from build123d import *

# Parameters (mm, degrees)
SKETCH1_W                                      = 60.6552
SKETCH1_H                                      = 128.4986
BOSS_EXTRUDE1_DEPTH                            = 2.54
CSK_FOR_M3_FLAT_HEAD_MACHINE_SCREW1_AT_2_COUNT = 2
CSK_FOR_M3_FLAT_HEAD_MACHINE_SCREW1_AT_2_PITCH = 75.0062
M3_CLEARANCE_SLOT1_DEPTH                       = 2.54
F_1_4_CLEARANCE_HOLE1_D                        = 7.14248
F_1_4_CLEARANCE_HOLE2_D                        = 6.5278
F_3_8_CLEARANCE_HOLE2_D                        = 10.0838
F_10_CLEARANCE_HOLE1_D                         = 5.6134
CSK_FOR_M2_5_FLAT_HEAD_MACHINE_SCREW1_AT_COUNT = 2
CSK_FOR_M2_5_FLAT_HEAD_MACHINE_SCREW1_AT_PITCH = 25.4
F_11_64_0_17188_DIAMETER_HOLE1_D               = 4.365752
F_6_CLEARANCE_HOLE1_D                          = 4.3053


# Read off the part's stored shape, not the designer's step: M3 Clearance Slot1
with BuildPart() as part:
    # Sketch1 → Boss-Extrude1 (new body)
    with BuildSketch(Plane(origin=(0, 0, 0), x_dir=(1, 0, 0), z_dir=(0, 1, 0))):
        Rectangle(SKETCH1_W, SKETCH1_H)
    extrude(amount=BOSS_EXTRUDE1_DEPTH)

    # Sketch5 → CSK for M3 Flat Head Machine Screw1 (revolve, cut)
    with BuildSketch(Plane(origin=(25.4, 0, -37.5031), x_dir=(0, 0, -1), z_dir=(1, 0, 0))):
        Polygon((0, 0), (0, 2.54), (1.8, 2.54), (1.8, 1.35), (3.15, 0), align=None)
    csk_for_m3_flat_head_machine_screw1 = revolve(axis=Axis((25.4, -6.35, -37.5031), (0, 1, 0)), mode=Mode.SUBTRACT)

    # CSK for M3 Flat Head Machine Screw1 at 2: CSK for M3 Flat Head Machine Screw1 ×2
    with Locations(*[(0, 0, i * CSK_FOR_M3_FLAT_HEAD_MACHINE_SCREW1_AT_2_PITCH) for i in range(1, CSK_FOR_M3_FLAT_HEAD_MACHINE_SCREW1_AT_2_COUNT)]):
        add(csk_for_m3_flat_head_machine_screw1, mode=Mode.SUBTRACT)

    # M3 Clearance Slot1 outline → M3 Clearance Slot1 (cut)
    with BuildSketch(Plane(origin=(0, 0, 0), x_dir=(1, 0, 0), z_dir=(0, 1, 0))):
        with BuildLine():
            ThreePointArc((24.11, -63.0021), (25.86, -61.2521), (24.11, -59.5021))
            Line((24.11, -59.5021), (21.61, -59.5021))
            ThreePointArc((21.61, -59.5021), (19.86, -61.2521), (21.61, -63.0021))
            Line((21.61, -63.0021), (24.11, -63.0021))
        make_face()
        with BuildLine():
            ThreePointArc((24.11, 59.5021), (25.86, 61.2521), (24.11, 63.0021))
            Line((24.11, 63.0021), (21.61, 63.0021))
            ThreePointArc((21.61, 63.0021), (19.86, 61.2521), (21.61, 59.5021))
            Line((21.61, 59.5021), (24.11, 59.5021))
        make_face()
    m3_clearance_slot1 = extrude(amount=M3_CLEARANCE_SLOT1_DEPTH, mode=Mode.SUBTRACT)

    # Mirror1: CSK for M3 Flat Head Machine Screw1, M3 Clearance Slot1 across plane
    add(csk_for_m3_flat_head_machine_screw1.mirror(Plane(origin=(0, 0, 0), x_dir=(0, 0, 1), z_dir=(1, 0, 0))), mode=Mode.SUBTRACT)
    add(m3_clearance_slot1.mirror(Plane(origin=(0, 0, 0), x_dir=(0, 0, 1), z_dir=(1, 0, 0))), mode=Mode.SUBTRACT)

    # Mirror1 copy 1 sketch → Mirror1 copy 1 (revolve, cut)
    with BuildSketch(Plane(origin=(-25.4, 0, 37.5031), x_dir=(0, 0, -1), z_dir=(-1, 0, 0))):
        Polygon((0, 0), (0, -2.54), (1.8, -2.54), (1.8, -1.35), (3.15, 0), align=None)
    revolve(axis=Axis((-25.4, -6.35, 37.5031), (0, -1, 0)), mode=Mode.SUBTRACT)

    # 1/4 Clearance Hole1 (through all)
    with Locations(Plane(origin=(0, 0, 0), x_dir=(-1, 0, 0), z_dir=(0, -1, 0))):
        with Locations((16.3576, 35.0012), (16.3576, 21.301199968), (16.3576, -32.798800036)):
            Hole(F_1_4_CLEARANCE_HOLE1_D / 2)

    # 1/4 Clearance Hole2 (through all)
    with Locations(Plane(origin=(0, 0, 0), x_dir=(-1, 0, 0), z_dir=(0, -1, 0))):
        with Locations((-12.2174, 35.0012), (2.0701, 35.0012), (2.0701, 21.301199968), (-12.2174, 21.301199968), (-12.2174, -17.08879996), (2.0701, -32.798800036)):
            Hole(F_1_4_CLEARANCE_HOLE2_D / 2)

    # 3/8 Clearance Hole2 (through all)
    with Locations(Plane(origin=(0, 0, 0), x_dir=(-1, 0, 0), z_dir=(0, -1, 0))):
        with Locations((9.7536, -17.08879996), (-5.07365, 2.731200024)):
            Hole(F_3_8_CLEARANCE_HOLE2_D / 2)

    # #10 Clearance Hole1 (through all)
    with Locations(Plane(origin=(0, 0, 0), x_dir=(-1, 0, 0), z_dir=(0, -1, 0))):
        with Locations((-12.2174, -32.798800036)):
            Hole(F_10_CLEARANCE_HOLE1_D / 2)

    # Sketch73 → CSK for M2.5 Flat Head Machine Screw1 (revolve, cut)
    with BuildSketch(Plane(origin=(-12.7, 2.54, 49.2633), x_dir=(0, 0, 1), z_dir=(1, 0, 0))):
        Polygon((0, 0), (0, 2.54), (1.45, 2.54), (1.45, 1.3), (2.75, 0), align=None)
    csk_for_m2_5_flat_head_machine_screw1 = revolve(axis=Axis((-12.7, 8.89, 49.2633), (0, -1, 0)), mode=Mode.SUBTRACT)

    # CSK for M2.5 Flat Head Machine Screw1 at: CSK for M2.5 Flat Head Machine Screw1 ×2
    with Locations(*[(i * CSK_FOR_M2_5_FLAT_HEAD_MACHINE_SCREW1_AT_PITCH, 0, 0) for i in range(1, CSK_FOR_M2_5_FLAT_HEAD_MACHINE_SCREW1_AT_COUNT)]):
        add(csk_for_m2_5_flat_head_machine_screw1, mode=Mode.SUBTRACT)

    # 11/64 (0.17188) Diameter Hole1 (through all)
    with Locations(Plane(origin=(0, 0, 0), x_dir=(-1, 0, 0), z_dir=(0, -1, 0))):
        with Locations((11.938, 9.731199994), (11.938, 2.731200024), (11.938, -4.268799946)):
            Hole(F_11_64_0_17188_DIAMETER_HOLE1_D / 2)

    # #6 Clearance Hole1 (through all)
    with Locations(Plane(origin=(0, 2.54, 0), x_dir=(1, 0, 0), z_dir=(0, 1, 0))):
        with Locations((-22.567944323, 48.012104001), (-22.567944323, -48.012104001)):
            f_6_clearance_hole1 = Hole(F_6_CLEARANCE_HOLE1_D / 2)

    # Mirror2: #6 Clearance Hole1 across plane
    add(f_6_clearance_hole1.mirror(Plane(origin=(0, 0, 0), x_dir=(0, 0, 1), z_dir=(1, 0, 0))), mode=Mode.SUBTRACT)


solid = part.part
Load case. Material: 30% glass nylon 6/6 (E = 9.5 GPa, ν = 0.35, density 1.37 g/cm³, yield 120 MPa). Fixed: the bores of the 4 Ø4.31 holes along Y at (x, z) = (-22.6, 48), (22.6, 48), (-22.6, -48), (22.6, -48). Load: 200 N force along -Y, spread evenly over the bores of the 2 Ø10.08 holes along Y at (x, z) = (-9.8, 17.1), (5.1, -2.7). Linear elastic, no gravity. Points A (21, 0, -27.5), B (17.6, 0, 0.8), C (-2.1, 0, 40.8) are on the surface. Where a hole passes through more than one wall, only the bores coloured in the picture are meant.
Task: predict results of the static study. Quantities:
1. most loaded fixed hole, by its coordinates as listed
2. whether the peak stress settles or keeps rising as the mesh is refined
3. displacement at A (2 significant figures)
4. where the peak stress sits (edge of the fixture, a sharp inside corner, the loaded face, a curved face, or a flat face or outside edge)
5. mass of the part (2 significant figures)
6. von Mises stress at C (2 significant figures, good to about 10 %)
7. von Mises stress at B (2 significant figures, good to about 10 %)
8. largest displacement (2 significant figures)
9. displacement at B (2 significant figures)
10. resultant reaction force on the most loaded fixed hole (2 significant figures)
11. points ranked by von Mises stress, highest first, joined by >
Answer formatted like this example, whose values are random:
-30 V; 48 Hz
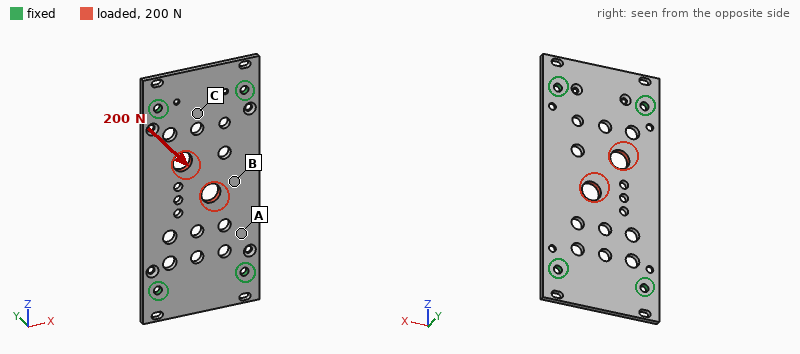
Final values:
(-22.6, 48); keeps rising; 0.46 mm; edge of the fixture; 24 g; 18 MPa; 29 MPa; 1.4 mm; 1.2 mm; 73 N; B > C > A
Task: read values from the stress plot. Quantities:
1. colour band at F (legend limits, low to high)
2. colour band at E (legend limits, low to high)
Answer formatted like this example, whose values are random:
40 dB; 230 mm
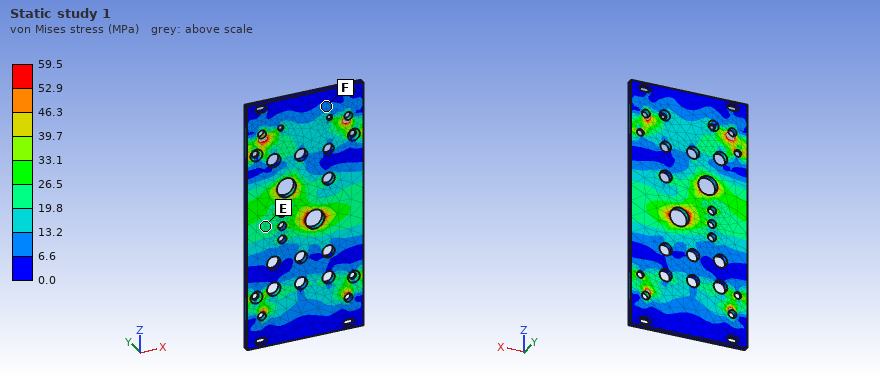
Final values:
6.6 to 13.2 MPa; 19.8 to 26.5 MPa
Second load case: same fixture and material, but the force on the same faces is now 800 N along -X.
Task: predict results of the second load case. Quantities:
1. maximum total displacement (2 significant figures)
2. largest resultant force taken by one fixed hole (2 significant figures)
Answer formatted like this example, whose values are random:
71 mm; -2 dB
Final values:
65 µm; 310 N
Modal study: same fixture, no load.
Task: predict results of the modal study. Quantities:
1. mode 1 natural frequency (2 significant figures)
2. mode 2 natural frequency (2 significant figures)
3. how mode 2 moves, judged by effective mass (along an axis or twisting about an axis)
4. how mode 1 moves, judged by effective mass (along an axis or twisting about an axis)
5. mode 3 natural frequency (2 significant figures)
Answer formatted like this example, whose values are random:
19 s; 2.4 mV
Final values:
700 Hz; 1000 Hz; twisting about Z; along Y; 1900 Hz
